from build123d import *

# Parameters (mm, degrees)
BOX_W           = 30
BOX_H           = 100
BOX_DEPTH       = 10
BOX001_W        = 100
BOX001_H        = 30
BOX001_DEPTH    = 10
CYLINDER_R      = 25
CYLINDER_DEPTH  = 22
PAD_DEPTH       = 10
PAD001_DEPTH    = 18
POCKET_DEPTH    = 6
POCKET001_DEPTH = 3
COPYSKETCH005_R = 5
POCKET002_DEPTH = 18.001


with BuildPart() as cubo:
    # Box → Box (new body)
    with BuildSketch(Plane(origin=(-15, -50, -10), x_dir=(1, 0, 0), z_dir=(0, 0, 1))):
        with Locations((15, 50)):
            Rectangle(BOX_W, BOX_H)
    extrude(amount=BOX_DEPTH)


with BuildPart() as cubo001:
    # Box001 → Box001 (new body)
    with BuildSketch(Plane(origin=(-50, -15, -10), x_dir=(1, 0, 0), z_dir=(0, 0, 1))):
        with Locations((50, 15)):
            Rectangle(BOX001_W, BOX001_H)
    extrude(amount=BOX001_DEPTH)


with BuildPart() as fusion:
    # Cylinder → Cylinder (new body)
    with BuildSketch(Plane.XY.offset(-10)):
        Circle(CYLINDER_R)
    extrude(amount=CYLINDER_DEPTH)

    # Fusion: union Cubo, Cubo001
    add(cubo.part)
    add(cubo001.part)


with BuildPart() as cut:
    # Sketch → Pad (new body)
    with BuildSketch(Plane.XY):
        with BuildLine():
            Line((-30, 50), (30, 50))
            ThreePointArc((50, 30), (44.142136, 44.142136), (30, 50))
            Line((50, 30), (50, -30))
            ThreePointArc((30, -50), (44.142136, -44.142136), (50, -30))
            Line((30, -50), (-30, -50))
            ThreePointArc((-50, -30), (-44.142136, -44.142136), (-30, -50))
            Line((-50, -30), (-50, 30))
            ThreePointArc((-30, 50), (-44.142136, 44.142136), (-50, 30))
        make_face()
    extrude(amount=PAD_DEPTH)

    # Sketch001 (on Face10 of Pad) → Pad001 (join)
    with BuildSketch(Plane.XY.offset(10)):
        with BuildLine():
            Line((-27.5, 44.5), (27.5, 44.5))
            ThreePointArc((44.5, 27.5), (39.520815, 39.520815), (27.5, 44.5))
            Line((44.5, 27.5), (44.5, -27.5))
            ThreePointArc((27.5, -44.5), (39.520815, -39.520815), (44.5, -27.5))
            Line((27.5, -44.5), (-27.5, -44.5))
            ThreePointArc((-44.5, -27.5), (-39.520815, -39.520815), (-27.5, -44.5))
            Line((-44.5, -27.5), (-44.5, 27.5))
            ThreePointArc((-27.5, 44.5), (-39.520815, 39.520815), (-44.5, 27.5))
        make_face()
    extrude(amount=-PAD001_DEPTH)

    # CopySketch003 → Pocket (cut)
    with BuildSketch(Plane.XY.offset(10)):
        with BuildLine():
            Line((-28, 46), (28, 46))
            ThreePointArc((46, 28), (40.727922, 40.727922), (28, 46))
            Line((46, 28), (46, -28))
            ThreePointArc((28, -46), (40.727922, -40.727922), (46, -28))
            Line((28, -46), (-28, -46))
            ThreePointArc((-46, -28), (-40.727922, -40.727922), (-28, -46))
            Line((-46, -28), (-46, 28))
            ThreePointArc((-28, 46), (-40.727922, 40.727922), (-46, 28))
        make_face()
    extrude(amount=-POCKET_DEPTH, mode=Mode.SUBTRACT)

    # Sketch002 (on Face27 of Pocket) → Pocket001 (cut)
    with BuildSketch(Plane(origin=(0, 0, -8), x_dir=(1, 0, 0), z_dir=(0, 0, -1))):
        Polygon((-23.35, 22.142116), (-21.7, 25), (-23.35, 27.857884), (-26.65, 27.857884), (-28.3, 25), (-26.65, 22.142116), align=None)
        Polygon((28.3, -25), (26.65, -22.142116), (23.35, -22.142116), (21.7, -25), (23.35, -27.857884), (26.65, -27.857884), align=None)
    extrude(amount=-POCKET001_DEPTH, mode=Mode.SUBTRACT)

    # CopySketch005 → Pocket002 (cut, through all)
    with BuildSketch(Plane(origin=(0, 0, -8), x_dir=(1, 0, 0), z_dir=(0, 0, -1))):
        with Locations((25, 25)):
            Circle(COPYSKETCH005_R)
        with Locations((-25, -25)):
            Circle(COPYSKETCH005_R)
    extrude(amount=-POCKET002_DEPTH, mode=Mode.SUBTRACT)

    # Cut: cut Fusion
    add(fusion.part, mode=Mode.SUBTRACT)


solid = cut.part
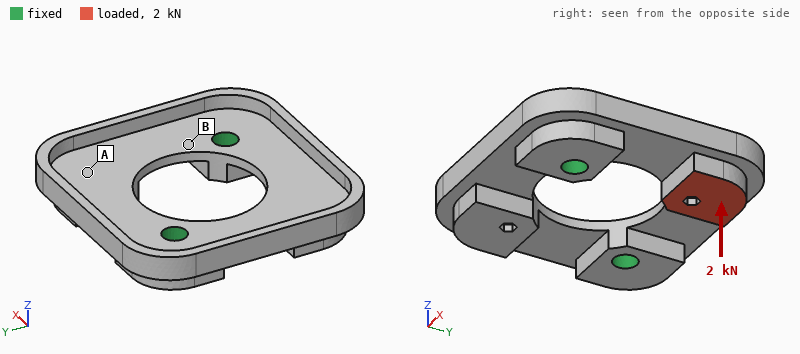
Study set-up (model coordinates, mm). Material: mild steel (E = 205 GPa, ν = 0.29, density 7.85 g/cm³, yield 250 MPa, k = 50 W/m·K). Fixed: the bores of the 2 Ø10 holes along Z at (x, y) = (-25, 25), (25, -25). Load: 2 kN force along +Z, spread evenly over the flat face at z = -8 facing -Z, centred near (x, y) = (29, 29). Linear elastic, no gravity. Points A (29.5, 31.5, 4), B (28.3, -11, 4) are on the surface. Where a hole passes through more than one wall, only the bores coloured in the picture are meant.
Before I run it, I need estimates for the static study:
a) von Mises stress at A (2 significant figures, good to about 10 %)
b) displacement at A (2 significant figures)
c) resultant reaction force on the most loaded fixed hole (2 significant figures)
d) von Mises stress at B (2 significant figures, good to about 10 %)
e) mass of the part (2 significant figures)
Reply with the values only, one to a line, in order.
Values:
25 MPa
0.16 mm
1.1 kN
110 MPa
490 g
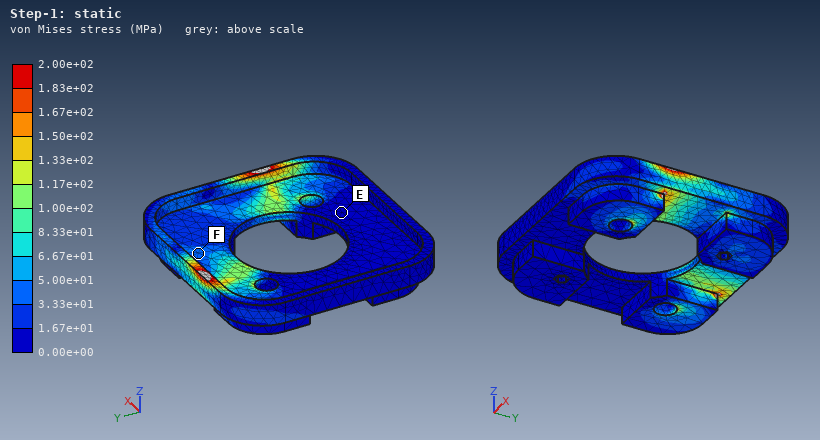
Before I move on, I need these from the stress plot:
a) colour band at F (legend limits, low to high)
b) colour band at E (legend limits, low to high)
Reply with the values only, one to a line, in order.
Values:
3.33e+01 to 5.00e+01 MPa
0.00e+00 to 1.67e+01 MPa
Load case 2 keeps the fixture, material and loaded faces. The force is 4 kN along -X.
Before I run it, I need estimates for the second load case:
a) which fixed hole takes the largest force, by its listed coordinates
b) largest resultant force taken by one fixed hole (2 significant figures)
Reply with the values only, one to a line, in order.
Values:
(-25, 25)
3.2 kN
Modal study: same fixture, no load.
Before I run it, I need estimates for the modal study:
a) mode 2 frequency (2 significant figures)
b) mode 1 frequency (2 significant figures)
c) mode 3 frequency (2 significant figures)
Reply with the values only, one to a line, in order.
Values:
1500 Hz
1500 Hz
5200 Hz
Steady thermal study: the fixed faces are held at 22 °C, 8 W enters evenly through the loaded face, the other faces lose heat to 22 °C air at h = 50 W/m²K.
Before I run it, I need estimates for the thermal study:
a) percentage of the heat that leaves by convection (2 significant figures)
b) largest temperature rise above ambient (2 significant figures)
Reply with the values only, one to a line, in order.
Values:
54 %
17 K
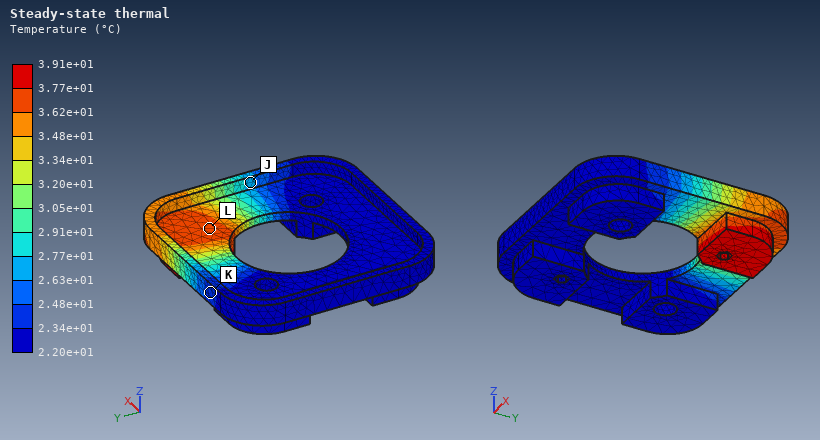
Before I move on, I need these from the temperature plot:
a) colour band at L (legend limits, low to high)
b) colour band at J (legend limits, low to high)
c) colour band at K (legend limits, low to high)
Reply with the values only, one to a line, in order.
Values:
3.62e+01 to 3.77e+01 °C
2.63e+01 to 2.77e+01 °C
2.34e+01 to 2.48e+01 °C
